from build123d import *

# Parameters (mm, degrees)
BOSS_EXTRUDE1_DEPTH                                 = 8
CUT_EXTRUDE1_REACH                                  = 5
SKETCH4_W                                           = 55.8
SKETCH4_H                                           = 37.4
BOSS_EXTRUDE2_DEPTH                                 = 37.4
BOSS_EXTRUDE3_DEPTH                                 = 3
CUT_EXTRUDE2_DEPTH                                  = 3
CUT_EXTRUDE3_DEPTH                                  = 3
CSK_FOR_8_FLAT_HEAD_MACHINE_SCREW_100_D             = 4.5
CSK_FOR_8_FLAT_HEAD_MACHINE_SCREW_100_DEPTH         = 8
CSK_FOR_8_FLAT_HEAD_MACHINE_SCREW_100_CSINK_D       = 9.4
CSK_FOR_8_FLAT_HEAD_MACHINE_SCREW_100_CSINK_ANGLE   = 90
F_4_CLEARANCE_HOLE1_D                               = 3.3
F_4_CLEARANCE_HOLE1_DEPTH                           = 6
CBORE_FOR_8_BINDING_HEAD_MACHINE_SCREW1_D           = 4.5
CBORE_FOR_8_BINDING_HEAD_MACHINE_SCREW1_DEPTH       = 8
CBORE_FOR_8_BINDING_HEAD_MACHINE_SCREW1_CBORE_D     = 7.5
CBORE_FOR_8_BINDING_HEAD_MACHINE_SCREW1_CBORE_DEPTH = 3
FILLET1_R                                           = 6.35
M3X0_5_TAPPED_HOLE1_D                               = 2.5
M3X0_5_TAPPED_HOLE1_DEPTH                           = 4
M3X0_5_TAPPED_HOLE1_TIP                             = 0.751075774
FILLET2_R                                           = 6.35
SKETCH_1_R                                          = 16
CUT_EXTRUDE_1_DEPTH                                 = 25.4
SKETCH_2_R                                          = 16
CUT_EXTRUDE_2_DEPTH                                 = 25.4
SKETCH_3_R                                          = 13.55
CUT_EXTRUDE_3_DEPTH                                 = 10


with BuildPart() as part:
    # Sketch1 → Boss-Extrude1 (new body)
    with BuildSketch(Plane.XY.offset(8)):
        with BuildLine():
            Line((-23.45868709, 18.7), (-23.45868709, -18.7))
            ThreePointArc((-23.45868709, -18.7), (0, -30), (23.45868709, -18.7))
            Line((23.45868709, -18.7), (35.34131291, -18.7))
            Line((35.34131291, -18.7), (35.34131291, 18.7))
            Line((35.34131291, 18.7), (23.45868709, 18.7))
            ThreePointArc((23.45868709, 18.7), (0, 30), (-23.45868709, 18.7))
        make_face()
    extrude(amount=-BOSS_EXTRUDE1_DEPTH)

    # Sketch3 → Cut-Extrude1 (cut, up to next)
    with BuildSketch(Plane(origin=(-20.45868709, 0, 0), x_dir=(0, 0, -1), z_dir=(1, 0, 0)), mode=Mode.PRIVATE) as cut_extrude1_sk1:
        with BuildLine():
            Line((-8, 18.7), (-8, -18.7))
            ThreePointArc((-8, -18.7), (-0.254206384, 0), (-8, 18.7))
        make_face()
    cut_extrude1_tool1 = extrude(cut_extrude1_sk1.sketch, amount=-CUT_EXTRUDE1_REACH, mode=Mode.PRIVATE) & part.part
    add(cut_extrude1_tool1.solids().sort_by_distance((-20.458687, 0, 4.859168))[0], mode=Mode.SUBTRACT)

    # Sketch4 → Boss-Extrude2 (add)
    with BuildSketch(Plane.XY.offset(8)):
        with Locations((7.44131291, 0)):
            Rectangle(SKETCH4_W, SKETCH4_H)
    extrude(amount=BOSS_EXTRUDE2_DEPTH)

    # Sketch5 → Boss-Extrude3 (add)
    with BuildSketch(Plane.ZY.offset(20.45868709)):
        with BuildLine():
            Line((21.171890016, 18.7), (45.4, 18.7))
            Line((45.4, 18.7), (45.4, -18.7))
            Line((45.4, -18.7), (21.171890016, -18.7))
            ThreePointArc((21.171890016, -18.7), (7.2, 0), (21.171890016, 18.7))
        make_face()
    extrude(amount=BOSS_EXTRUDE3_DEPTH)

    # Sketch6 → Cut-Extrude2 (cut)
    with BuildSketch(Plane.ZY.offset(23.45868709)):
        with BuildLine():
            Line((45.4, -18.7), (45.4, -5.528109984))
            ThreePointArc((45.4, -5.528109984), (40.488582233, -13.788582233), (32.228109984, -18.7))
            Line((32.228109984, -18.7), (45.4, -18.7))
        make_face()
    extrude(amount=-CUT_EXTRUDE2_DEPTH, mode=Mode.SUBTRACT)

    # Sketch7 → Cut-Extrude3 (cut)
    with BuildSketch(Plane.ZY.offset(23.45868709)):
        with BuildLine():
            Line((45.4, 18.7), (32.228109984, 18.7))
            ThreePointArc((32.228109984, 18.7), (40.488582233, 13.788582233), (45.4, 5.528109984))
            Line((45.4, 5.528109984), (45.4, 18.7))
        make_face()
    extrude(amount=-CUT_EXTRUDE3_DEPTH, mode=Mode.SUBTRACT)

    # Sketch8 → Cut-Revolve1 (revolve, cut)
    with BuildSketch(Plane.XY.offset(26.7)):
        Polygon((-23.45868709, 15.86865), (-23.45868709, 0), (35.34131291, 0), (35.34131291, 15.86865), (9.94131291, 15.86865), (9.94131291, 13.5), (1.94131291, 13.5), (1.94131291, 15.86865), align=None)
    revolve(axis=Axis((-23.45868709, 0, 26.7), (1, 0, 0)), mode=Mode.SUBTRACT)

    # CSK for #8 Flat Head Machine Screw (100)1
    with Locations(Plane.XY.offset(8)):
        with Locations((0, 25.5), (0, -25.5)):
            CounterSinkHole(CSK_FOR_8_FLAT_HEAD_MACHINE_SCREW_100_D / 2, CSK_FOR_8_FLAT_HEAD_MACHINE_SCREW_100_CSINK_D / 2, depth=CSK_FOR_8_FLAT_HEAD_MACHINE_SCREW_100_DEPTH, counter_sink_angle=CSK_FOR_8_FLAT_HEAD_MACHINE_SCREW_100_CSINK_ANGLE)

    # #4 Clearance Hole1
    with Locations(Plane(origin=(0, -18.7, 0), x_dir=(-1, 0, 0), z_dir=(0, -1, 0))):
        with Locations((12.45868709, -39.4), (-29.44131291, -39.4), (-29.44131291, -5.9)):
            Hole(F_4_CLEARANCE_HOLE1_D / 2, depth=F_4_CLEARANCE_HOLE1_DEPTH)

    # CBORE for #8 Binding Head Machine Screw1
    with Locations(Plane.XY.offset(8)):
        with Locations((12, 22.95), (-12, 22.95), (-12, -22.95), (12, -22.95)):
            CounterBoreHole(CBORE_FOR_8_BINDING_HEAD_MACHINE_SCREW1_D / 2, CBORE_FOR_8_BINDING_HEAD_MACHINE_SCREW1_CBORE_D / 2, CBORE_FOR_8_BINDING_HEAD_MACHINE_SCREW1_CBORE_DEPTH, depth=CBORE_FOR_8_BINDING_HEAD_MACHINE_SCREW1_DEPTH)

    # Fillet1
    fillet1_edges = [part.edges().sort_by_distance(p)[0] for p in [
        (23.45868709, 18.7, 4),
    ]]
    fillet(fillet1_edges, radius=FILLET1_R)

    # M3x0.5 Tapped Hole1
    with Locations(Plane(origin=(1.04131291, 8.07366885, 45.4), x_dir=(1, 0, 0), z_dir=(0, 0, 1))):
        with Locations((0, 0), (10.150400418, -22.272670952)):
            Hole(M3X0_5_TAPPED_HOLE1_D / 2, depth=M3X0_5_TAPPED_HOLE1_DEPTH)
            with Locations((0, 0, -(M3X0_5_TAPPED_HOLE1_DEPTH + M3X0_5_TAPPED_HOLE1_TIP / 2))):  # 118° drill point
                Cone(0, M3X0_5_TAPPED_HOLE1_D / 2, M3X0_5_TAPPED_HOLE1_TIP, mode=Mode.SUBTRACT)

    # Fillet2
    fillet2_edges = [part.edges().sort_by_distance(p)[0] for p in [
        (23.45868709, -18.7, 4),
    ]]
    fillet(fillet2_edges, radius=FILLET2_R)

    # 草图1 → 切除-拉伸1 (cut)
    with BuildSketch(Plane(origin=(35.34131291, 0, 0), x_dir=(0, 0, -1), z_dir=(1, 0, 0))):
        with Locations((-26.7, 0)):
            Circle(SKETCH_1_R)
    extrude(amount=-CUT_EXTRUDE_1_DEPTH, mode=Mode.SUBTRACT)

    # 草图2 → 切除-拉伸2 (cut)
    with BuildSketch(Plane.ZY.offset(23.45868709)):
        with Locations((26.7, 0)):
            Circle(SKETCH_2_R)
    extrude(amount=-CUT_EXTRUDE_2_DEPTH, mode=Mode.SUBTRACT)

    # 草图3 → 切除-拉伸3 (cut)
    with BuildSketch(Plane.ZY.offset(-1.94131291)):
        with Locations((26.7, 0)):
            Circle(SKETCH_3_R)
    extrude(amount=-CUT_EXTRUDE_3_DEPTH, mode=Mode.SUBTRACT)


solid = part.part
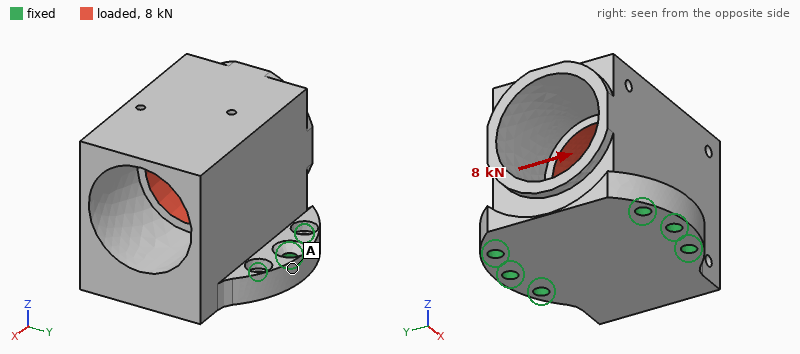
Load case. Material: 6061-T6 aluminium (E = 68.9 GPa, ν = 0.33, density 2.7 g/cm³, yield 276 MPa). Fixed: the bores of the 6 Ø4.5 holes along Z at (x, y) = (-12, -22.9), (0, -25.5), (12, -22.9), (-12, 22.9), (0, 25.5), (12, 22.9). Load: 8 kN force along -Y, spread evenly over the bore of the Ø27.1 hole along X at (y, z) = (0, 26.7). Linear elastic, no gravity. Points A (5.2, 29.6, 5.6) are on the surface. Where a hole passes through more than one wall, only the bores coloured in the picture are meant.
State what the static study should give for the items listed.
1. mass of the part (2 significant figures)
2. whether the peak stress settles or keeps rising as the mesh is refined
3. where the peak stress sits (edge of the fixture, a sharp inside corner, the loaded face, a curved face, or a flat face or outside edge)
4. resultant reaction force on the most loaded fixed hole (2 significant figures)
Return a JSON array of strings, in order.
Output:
["160 g", "keeps rising", "edge of the fixture", "2.6 kN"]
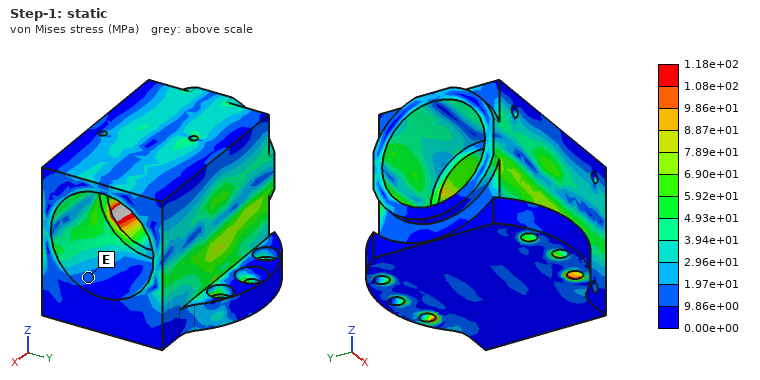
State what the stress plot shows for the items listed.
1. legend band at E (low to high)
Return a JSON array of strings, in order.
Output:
["9.86e+00 to 1.97e+01 MPa"]
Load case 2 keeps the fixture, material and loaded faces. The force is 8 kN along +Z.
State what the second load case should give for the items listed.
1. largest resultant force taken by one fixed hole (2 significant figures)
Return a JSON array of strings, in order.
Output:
["2.6 kN"]
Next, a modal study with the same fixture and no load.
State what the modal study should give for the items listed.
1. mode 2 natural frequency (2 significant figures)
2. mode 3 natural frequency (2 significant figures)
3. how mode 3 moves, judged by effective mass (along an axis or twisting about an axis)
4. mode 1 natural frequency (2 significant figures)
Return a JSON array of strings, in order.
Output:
["4800 Hz", "8100 Hz", "twisting about Z", "4800 Hz"]
